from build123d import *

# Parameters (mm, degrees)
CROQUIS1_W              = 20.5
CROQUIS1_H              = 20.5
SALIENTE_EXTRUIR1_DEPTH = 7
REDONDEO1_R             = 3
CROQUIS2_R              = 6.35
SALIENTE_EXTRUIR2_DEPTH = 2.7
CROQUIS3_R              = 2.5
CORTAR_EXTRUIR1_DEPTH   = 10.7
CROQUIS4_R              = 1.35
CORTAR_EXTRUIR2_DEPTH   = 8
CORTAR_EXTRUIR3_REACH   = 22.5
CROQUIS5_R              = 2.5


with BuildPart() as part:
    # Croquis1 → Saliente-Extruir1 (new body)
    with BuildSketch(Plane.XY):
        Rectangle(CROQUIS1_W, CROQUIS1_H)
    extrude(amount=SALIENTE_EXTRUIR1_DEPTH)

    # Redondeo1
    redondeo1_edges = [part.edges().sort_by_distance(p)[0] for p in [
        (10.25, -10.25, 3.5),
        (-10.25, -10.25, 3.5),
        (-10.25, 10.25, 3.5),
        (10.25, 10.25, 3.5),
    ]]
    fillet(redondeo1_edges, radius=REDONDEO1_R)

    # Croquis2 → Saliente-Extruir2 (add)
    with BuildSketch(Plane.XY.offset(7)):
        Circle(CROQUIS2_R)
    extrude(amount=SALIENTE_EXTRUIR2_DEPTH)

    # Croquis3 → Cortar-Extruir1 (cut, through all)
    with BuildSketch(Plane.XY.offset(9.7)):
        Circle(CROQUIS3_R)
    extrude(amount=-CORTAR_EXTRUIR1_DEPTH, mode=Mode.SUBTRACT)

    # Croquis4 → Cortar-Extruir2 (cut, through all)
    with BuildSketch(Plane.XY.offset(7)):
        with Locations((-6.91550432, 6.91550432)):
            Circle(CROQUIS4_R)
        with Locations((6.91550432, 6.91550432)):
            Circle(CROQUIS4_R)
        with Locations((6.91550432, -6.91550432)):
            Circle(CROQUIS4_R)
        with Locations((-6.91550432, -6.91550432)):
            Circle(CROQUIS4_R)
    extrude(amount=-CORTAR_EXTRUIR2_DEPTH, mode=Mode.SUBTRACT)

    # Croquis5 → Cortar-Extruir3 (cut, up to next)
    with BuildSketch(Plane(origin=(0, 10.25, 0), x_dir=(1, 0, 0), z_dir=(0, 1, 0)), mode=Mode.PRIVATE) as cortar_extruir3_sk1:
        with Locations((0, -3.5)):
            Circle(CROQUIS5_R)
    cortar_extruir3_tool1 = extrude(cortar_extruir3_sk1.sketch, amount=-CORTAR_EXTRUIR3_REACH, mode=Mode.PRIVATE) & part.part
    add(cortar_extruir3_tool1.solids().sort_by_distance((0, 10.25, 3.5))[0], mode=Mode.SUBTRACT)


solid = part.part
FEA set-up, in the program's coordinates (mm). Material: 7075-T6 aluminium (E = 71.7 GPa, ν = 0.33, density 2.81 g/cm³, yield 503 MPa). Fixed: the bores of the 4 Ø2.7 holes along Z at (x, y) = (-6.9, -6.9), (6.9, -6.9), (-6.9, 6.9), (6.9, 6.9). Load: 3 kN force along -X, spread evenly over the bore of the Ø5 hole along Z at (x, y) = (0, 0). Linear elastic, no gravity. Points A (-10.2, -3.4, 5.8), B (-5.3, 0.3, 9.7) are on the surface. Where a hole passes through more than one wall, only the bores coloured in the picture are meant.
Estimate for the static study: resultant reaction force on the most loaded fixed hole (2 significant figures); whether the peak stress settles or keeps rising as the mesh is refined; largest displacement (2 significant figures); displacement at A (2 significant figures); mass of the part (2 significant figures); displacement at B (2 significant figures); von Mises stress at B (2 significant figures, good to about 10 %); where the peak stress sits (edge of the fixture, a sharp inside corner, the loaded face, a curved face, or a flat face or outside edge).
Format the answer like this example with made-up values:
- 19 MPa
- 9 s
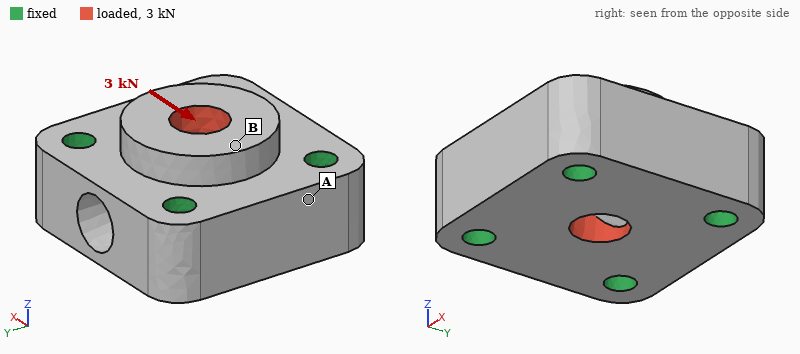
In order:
- 970 N
- keeps rising
- 4.8 µm
- 1.6 µm
- 7.6 g
- 4.0 µm
- 21 MPa
- edge of the fixture
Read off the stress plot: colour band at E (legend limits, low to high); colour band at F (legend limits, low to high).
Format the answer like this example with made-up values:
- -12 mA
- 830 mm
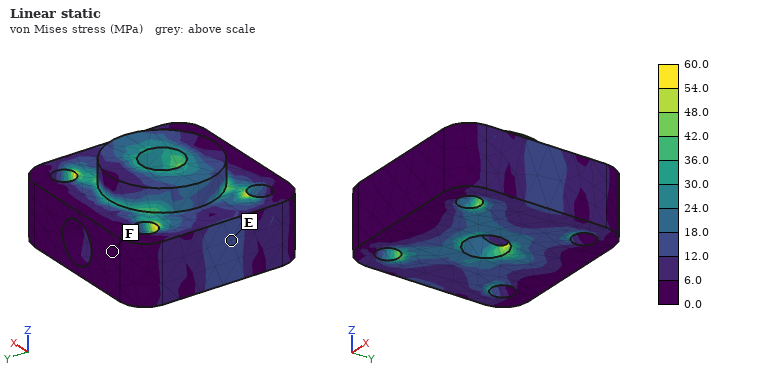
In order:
- 12.0 to 18.0 MPa
- 0.0 to 6.0 MPa
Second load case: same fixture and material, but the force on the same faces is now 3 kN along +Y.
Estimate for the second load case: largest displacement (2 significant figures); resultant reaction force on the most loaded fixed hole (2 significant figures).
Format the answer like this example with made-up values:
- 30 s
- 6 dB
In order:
- 4.7 µm
- 890 N
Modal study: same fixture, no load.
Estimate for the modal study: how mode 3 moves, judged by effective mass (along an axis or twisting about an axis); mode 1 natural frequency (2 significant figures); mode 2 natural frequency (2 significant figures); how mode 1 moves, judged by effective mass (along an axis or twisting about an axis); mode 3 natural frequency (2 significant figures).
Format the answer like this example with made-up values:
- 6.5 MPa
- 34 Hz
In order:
- along Y
- 81 kHz
- 93 kHz
- along Z
- 97 kHz
